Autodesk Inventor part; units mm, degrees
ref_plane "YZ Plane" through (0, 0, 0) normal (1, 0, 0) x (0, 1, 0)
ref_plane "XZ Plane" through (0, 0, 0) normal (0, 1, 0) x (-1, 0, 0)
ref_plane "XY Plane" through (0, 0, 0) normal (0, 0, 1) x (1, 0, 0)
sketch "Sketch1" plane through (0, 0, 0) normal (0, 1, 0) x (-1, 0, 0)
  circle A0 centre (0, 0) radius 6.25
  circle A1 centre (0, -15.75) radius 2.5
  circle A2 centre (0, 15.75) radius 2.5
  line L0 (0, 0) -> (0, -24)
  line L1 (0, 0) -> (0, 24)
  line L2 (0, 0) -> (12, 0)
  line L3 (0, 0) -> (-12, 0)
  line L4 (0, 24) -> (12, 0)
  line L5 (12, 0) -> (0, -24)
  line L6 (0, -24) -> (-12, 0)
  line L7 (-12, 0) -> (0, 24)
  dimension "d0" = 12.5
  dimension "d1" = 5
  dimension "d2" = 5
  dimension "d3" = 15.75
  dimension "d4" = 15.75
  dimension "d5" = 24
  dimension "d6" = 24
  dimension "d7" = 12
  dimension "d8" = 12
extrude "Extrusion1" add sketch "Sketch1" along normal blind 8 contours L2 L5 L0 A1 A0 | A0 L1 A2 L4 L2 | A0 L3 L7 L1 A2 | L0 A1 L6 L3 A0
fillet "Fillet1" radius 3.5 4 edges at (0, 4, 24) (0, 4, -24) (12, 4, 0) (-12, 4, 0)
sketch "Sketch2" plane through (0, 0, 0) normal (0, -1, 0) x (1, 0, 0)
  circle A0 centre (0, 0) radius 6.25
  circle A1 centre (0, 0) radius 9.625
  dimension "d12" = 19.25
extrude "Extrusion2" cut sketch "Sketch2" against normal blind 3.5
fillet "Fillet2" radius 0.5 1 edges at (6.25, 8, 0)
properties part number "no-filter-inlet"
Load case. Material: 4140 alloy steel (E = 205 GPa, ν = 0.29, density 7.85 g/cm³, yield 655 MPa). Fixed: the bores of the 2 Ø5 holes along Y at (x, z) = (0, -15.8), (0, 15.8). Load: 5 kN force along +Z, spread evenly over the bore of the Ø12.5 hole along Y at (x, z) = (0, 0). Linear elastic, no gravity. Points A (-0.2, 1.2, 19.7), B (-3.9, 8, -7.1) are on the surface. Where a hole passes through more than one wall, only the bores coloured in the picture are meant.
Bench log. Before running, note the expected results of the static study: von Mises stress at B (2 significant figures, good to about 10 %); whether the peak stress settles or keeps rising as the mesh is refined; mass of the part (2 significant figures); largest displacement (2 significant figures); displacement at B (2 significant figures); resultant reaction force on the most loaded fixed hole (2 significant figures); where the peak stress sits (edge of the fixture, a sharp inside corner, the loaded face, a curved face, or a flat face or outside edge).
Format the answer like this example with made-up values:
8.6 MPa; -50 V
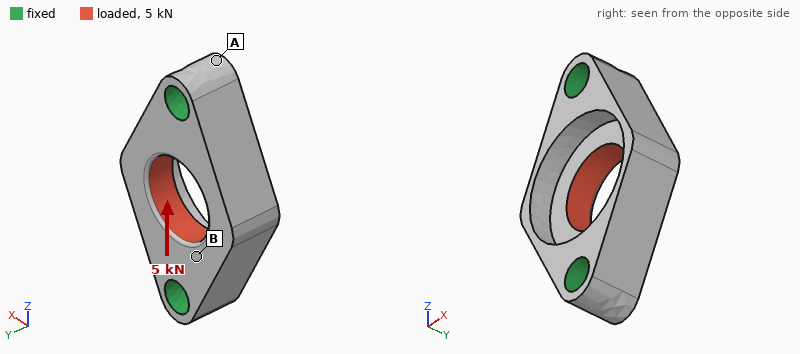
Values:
45 MPa; keeps rising; 20 g; 3.5 µm; 1.9 µm; 2.5 kN; edge of the fixture
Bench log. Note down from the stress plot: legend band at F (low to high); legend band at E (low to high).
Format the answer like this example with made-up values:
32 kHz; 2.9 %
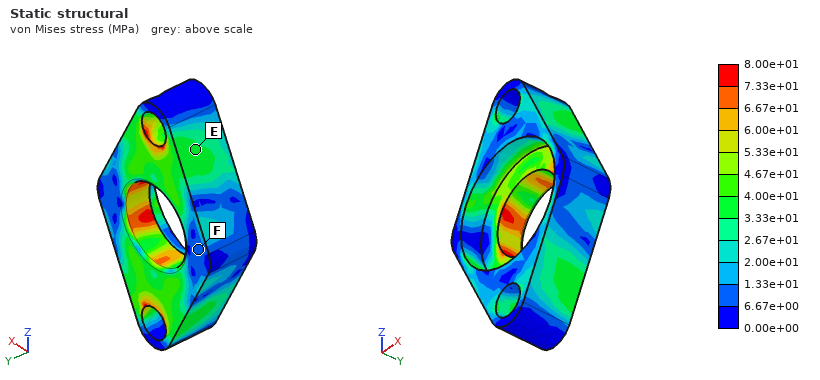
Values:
6.67e+00 to 1.33e+01 MPa; 3.33e+01 to 4.00e+01 MPa
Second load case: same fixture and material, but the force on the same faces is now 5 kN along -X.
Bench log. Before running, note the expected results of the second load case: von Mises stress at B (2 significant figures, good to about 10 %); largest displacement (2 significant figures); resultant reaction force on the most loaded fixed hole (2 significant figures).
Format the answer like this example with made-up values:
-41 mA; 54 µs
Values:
56 MPa; 8.4 µm; 2.5 kN
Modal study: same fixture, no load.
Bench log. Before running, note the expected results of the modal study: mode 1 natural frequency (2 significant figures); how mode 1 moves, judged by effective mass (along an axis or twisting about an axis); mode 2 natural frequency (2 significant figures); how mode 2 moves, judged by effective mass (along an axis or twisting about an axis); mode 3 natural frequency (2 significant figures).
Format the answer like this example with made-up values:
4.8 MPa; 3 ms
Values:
28 kHz; twisting about Z; 30 kHz; along Y; 48 kHz
